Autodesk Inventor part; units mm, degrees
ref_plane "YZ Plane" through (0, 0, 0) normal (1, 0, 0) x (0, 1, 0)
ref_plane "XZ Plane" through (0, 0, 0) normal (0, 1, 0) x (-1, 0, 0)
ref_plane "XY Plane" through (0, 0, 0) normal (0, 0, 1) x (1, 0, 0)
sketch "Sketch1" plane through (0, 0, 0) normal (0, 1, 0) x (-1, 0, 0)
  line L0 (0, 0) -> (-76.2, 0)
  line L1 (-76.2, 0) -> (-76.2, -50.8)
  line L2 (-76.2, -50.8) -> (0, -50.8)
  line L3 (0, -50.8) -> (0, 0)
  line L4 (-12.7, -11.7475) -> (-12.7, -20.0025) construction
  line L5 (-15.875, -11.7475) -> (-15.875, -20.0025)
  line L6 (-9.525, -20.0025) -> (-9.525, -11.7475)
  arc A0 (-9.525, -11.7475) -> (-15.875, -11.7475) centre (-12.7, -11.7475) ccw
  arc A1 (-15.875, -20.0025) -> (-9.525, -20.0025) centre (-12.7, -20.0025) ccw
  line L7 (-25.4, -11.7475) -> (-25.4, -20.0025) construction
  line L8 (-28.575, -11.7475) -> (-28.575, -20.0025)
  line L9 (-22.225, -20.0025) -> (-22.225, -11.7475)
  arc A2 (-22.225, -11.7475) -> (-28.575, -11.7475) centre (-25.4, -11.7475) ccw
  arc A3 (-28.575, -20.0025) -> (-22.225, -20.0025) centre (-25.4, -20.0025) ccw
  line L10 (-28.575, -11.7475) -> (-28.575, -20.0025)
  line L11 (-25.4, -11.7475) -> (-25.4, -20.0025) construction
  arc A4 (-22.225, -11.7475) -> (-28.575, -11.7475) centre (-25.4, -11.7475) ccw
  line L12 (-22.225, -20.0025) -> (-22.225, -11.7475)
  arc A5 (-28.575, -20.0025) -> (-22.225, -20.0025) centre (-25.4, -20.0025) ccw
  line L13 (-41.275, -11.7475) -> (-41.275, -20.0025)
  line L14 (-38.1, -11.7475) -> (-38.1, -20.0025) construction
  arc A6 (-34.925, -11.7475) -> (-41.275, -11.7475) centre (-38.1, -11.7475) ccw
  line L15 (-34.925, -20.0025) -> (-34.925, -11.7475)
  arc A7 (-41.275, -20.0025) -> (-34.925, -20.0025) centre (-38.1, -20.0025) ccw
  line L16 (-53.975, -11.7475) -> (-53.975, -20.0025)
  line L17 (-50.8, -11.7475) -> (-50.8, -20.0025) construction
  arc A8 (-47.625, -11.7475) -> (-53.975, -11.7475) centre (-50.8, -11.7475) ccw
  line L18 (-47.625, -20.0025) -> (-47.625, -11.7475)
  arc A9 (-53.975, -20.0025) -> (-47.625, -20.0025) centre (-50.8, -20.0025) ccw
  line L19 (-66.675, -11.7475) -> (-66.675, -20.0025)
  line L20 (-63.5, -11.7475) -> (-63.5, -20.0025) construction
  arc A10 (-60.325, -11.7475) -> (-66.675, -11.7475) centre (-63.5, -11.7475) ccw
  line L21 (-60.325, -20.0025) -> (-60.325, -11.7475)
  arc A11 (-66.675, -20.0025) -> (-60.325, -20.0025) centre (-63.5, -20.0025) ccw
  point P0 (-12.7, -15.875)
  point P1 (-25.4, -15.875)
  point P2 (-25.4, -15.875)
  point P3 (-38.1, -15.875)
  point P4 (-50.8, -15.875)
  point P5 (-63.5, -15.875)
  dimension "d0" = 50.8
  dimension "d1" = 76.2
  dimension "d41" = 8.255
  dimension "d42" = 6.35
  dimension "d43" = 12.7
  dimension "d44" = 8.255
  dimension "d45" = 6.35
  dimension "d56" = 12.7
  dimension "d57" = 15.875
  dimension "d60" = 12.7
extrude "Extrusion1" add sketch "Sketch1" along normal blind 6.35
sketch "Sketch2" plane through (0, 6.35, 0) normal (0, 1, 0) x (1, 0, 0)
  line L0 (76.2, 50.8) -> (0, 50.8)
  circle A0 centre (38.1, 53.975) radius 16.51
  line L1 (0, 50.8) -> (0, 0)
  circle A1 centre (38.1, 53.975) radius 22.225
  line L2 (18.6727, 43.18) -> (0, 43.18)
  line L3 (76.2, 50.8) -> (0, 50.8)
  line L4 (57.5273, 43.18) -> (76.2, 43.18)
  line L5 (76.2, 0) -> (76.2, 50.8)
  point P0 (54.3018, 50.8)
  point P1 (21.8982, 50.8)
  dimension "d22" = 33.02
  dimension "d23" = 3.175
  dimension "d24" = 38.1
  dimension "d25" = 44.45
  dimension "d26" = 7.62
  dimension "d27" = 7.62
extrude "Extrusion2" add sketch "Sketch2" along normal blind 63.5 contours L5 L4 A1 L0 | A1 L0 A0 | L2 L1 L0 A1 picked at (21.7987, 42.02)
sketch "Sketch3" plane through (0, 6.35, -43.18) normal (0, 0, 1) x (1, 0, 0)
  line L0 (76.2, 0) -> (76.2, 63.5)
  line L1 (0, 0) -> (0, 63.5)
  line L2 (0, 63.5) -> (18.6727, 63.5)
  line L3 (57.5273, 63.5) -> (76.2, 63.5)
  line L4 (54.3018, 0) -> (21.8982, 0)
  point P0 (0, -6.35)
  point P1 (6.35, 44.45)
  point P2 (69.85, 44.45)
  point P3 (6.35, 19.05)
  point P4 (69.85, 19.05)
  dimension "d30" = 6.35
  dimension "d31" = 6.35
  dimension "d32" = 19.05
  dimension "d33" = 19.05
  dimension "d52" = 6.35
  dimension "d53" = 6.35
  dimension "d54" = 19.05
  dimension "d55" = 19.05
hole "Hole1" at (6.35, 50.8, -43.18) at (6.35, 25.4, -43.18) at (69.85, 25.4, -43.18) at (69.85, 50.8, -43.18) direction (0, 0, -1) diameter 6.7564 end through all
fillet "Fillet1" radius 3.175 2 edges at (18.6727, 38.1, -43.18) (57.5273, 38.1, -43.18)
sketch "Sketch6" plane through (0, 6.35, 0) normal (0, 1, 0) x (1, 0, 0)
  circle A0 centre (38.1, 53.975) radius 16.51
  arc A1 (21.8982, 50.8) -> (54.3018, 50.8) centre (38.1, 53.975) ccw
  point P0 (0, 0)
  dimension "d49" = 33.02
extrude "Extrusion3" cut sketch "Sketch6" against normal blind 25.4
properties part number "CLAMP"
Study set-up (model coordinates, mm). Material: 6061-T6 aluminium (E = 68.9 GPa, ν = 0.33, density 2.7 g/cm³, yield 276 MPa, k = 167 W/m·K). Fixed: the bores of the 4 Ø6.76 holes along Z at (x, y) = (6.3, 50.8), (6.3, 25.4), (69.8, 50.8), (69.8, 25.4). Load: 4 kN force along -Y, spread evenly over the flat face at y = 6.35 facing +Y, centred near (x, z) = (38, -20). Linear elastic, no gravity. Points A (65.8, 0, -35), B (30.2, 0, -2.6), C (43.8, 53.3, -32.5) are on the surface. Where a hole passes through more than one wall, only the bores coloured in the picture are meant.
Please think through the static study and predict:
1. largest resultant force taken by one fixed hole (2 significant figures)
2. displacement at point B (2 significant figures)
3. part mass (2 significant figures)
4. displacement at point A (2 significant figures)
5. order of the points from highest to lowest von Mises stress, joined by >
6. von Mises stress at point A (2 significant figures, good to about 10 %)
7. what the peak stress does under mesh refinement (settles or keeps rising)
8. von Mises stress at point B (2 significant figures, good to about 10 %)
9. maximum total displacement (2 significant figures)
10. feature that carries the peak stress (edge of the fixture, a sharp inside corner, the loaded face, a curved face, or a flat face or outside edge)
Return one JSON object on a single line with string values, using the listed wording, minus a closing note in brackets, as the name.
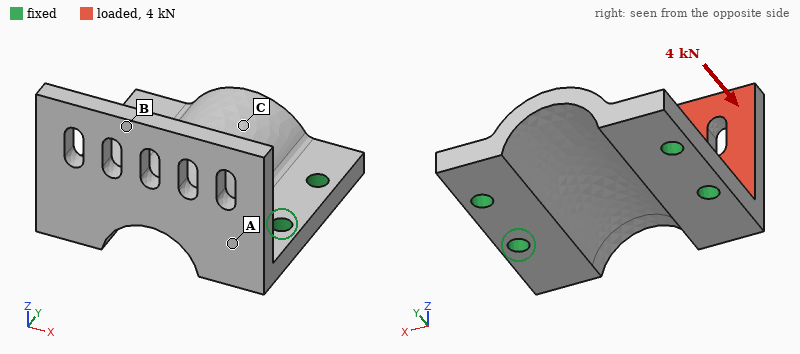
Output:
{"largest resultant force taken by one fixed hole": "2.4 kN", "displacement at point B": "0.49 mm", "part mass": "150 g", "displacement at point A": "0.14 mm", "order of the points from highest to lowest von Mises stress, joined by >": "A > B > C", "von Mises stress at point A": "76 MPa", "what the peak stress does under mesh refinement": "keeps rising", "von Mises stress at point B": "35 MPa", "maximum total displacement": "0.60 mm", "feature that carries the peak stress": "edge of the fixture"}
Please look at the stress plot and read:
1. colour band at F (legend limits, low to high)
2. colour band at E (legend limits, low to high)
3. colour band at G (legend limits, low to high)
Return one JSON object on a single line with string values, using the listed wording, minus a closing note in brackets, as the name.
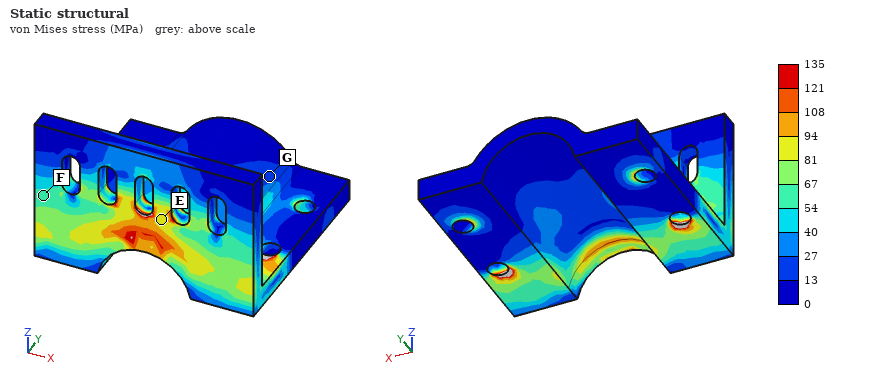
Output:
{"colour band at F": "54 to 67 MPa", "colour band at E": "81 to 94 MPa", "colour band at G": "13 to 27 MPa"}
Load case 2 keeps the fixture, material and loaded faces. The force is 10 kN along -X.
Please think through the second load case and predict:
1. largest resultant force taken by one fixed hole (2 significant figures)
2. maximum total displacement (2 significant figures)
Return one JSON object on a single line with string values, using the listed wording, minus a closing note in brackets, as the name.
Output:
{"largest resultant force taken by one fixed hole": "6.2 kN", "maximum total displacement": "0.36 mm"}
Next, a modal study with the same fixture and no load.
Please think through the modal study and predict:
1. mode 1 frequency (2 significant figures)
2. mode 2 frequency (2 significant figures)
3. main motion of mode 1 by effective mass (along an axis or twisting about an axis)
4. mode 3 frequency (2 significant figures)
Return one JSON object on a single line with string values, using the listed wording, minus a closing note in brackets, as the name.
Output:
{"mode 1 frequency": "2400 Hz", "mode 2 frequency": "3400 Hz", "main motion of mode 1 by effective mass": "along Y", "mode 3 frequency": "5500 Hz"}
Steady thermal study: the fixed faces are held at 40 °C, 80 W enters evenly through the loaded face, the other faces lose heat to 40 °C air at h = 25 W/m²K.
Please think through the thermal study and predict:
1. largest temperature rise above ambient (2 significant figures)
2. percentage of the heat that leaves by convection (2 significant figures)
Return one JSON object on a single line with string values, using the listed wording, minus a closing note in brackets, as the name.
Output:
{"largest temperature rise above ambient": "45 K", "percentage of the heat that leaves by convection": "8.5 %"}
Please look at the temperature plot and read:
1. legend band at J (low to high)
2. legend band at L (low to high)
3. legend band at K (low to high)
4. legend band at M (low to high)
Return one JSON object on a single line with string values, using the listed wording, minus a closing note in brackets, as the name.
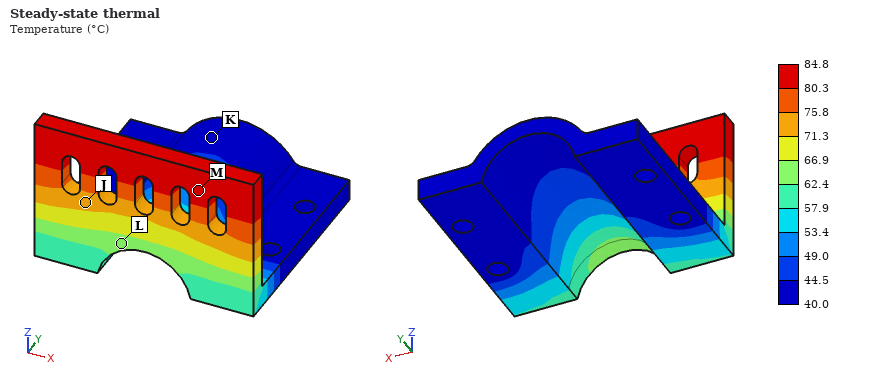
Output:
{"legend band at J": "71.3 to 75.8 °C", "legend band at L": "62.4 to 66.9 °C", "legend band at K": "40.0 to 44.5 °C", "legend band at M": "80.3 to 84.8 °C"}
